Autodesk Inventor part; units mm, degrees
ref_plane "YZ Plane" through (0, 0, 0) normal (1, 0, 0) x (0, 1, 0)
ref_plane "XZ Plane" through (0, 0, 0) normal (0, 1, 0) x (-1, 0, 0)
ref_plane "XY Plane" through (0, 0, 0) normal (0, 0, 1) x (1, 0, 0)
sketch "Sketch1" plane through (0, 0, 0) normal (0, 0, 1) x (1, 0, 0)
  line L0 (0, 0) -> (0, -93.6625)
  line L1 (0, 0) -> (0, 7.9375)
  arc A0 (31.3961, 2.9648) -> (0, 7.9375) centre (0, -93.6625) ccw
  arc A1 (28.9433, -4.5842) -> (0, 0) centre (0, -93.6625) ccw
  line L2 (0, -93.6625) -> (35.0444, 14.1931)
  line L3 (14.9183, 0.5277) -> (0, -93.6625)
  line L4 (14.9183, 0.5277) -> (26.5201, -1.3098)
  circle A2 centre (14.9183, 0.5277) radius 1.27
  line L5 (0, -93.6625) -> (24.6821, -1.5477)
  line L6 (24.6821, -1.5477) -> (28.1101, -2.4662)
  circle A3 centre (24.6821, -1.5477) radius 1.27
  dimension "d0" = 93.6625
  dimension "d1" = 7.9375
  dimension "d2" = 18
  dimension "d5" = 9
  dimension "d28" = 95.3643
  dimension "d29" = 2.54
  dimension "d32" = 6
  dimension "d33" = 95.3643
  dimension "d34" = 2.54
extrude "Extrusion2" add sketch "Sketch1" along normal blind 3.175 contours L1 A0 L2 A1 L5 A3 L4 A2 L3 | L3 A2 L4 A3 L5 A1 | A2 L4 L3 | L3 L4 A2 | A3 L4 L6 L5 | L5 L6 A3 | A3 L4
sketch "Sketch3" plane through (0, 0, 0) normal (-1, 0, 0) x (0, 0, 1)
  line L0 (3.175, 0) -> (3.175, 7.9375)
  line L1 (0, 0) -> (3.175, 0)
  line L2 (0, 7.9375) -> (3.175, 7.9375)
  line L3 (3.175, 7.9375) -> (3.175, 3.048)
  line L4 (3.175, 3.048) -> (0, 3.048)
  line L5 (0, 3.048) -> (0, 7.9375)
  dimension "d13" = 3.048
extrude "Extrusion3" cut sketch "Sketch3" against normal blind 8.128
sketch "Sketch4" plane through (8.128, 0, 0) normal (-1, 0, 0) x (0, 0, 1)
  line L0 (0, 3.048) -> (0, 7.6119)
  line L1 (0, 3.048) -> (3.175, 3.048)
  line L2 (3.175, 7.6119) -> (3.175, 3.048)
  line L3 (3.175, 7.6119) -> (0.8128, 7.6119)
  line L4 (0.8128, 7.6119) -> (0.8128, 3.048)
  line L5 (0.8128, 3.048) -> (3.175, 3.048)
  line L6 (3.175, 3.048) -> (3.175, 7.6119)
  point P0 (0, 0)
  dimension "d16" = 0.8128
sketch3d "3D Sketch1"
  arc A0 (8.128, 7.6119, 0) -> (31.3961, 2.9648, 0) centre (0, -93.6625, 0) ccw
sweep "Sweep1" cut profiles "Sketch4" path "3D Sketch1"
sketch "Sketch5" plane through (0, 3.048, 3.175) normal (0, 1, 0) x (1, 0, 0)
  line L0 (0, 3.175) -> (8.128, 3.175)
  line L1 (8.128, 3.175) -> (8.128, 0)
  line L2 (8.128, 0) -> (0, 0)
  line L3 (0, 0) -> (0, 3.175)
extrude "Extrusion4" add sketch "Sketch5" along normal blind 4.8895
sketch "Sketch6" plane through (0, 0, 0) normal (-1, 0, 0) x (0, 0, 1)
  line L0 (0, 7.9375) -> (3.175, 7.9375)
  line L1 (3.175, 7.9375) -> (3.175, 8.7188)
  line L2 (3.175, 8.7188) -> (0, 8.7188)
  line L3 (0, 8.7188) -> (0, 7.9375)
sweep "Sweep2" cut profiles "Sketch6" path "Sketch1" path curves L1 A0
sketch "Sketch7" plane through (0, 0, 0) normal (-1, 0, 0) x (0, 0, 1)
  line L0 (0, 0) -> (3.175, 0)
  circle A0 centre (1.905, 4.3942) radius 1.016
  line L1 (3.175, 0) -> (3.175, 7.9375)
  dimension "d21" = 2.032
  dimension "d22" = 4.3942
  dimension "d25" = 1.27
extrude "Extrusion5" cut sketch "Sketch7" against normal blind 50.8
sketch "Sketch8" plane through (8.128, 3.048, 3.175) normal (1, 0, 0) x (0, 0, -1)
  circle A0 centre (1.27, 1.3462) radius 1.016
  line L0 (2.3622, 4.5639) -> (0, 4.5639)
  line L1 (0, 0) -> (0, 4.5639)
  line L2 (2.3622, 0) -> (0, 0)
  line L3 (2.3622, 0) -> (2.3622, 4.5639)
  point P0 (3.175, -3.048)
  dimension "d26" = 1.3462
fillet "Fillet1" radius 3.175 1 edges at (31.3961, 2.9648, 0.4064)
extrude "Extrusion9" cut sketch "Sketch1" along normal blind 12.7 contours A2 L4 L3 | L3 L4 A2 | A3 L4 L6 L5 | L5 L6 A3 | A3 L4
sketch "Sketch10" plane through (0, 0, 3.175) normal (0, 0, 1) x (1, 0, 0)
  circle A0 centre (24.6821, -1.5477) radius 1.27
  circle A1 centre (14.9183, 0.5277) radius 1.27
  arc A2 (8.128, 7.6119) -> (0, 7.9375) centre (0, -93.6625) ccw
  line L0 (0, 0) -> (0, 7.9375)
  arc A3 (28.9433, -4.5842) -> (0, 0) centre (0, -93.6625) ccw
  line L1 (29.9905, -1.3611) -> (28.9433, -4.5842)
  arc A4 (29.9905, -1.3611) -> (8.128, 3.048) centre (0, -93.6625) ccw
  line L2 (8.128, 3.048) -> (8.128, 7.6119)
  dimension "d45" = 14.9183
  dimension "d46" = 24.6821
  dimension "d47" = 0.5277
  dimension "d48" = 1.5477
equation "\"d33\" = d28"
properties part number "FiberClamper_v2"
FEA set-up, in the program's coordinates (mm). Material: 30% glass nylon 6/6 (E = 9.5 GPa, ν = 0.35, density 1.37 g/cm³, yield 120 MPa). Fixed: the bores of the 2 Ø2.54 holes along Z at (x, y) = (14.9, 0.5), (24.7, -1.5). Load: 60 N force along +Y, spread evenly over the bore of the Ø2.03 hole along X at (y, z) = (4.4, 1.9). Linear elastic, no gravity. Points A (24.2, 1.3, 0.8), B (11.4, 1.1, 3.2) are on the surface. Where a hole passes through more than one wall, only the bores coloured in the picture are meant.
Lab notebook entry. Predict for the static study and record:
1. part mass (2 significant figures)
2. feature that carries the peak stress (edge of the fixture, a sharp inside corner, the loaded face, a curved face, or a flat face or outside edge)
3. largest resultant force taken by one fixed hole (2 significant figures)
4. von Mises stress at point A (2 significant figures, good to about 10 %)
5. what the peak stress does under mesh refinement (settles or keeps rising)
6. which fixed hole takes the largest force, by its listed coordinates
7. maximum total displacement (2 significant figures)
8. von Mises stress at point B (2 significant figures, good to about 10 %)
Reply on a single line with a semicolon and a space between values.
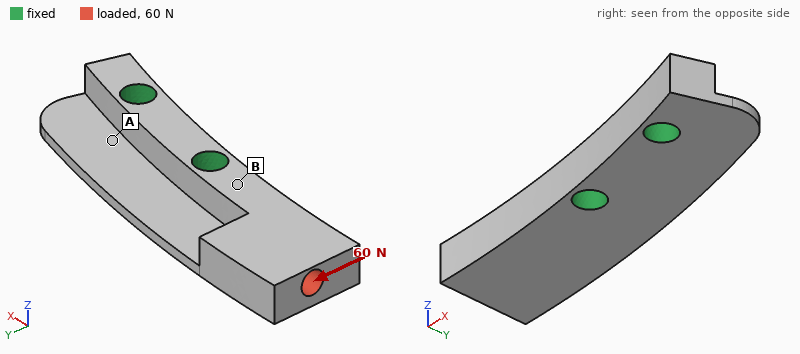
0.64 g; edge of the fixture; 92 N; 7.3 MPa; keeps rising; (14.9, 0.5); 0.16 mm; 19 MPa
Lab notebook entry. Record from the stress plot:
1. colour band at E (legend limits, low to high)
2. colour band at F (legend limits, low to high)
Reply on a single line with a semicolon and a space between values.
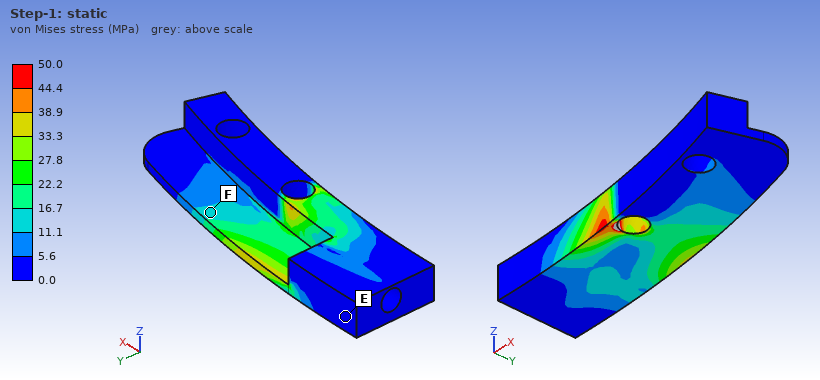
0.0 to 5.6 MPa; 11.1 to 16.7 MPa
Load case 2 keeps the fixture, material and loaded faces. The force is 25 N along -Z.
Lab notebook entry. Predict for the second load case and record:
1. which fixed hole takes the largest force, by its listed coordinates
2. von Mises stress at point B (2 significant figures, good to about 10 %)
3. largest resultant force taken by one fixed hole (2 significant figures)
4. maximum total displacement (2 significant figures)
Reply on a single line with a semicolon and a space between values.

(14.9, 0.5); 35 MPa; 26 N; 0.20 mm
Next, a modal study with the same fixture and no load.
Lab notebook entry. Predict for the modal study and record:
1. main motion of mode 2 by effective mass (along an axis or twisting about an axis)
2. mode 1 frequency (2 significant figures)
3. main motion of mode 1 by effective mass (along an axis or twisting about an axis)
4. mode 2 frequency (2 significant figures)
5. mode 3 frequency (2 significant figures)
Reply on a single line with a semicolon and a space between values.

along Y; 4500 Hz; along Z; 7600 Hz; 11 kHz
